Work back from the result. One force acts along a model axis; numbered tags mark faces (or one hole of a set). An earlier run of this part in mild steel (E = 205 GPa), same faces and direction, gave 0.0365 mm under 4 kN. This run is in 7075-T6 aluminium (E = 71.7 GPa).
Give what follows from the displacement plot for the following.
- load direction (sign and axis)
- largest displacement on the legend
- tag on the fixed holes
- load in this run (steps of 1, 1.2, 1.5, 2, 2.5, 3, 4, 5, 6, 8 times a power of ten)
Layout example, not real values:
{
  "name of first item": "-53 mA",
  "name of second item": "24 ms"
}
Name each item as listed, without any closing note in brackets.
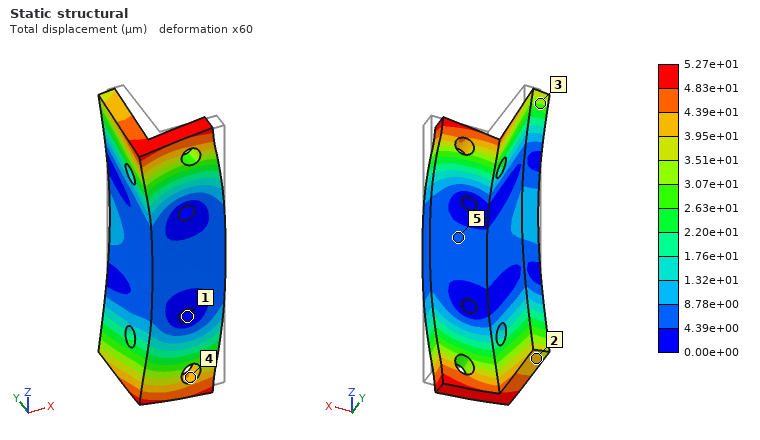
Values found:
{
  "load direction": "-X",
  "largest displacement on the legend": "5.27e+01 µm",
  "tag on the fixed holes": "1",
  "load in this run": "2 kN"
}
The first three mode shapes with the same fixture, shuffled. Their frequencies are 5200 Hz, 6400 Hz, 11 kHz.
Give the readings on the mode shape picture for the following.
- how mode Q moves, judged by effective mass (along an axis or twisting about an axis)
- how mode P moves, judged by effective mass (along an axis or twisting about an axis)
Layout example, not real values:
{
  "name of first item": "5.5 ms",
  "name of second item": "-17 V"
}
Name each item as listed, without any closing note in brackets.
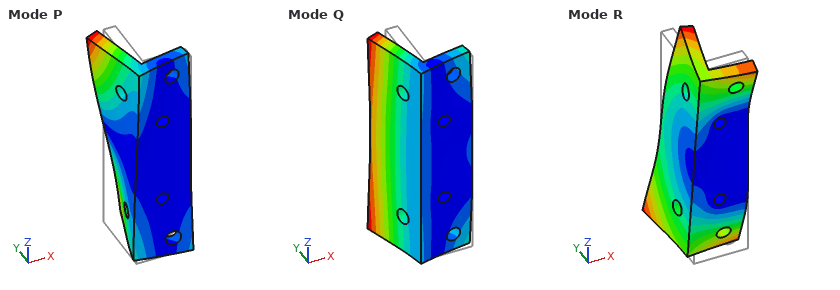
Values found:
{
  "how mode Q moves, judged by effective mass": "along X",
  "how mode P moves, judged by effective mass": "twisting about Y"
}
